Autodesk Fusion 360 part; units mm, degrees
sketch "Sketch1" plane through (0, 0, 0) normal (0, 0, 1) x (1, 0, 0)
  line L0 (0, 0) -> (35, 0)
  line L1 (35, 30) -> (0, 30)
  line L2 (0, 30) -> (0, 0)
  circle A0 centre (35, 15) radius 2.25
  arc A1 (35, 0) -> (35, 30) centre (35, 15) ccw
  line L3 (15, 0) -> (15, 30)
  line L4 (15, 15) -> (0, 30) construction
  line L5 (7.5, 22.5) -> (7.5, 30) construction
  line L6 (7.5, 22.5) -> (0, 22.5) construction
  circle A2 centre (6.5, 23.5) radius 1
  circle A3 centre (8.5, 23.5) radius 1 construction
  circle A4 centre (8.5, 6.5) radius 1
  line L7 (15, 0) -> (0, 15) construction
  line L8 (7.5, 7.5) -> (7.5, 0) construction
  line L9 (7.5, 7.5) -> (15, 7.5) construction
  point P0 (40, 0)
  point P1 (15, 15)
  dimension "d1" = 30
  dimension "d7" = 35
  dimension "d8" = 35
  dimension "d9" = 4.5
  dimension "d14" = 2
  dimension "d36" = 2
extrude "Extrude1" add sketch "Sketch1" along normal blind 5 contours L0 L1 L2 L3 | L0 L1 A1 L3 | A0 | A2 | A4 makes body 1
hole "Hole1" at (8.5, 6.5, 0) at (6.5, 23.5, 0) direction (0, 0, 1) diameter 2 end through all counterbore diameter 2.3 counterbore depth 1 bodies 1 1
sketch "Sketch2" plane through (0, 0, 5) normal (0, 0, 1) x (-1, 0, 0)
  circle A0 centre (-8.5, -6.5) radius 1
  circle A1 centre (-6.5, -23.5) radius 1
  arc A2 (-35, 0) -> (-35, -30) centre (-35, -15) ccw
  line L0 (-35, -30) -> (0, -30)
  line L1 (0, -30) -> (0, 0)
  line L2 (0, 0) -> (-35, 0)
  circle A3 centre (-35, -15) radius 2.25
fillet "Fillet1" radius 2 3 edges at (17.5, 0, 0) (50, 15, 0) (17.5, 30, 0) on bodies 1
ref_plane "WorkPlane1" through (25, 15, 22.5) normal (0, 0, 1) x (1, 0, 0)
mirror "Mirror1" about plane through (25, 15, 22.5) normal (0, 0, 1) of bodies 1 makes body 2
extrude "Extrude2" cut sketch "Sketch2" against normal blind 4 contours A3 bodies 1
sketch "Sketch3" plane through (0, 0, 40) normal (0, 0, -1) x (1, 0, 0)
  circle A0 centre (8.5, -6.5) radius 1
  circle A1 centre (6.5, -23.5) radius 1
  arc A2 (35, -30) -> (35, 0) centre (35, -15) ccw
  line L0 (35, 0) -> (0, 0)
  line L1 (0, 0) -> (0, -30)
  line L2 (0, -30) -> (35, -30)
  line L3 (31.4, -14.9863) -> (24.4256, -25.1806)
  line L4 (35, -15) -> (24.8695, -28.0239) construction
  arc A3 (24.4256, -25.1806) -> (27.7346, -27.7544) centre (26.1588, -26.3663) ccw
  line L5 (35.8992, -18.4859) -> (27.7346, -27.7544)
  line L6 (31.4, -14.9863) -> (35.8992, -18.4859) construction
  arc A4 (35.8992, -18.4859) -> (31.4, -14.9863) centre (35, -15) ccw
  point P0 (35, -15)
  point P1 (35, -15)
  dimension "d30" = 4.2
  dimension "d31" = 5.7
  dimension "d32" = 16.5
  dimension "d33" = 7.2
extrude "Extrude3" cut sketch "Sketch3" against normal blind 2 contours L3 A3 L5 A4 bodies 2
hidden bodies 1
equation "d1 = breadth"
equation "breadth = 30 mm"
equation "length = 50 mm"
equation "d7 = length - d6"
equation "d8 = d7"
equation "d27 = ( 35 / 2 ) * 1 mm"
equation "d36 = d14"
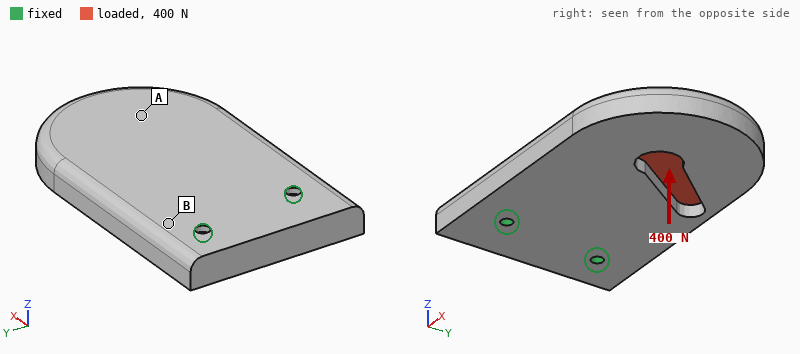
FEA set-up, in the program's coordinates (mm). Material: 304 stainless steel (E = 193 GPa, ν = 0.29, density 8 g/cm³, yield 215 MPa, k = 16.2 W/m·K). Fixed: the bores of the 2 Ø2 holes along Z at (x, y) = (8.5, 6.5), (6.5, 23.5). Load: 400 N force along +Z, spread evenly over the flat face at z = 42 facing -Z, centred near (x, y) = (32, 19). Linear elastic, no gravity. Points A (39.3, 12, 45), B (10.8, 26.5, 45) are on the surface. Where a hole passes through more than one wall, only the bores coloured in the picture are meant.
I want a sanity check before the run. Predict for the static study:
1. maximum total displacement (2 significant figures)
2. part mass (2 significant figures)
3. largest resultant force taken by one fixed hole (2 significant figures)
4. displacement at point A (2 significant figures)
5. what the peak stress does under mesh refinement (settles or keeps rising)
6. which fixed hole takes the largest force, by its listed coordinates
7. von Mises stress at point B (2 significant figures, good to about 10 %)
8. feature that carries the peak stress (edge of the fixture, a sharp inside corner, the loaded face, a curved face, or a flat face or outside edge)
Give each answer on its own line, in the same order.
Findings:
97 µm
53 g
230 N
66 µm
keeps rising
(6.5, 23.5)
68 MPa
edge of the fixture
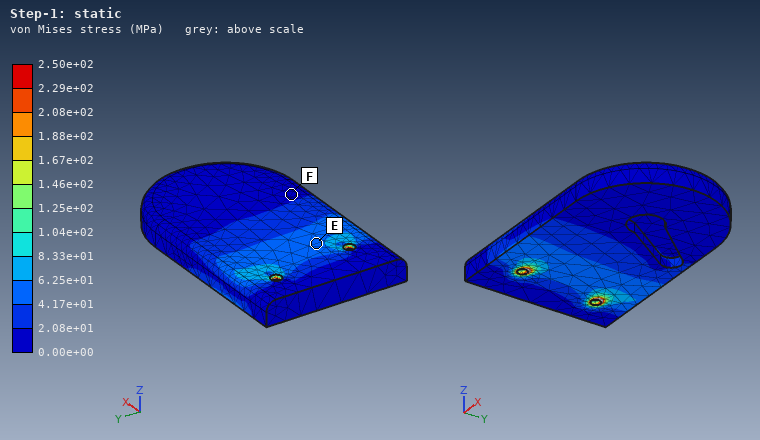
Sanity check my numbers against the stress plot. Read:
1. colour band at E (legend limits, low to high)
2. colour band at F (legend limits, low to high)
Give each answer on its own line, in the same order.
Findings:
4.17e+01 to 6.25e+01 MPa
0.00e+00 to 2.08e+01 MPa
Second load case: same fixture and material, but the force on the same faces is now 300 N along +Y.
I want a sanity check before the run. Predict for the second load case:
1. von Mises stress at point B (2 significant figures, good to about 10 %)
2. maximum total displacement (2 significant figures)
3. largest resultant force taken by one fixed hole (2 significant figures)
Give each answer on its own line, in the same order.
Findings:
6.3 MPa
3.5 µm
440 N
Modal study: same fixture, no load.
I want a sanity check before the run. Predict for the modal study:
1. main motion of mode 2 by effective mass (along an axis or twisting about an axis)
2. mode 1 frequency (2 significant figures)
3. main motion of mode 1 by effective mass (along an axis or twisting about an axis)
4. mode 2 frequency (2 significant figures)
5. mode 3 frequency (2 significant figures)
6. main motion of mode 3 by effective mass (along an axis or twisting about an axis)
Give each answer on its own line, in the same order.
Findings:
twisting about X
2200 Hz
along Z
7300 Hz
9500 Hz
along Y
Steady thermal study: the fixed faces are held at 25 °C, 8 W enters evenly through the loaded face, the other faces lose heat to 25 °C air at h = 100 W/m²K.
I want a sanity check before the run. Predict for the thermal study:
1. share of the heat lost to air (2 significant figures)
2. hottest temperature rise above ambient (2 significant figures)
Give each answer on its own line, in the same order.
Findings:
73 %
47 K
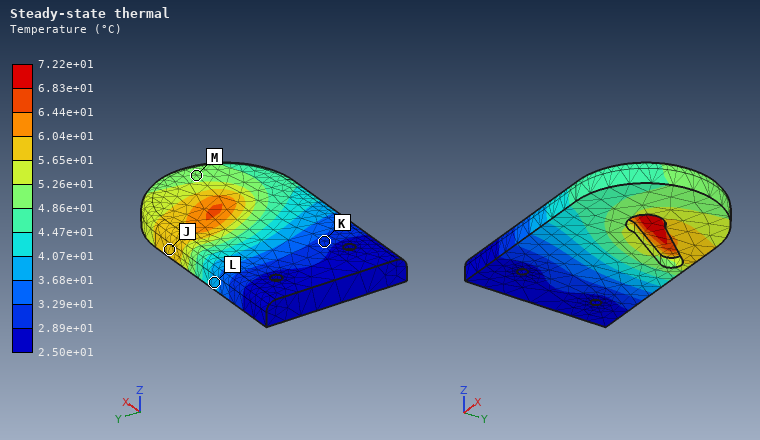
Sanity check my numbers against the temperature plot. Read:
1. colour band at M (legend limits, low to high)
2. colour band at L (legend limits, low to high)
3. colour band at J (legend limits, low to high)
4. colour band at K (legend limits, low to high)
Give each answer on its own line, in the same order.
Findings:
4.86e+01 to 5.26e+01 °C
3.68e+01 to 4.07e+01 °C
5.65e+01 to 6.04e+01 °C
2.89e+01 to 3.29e+01 °C
